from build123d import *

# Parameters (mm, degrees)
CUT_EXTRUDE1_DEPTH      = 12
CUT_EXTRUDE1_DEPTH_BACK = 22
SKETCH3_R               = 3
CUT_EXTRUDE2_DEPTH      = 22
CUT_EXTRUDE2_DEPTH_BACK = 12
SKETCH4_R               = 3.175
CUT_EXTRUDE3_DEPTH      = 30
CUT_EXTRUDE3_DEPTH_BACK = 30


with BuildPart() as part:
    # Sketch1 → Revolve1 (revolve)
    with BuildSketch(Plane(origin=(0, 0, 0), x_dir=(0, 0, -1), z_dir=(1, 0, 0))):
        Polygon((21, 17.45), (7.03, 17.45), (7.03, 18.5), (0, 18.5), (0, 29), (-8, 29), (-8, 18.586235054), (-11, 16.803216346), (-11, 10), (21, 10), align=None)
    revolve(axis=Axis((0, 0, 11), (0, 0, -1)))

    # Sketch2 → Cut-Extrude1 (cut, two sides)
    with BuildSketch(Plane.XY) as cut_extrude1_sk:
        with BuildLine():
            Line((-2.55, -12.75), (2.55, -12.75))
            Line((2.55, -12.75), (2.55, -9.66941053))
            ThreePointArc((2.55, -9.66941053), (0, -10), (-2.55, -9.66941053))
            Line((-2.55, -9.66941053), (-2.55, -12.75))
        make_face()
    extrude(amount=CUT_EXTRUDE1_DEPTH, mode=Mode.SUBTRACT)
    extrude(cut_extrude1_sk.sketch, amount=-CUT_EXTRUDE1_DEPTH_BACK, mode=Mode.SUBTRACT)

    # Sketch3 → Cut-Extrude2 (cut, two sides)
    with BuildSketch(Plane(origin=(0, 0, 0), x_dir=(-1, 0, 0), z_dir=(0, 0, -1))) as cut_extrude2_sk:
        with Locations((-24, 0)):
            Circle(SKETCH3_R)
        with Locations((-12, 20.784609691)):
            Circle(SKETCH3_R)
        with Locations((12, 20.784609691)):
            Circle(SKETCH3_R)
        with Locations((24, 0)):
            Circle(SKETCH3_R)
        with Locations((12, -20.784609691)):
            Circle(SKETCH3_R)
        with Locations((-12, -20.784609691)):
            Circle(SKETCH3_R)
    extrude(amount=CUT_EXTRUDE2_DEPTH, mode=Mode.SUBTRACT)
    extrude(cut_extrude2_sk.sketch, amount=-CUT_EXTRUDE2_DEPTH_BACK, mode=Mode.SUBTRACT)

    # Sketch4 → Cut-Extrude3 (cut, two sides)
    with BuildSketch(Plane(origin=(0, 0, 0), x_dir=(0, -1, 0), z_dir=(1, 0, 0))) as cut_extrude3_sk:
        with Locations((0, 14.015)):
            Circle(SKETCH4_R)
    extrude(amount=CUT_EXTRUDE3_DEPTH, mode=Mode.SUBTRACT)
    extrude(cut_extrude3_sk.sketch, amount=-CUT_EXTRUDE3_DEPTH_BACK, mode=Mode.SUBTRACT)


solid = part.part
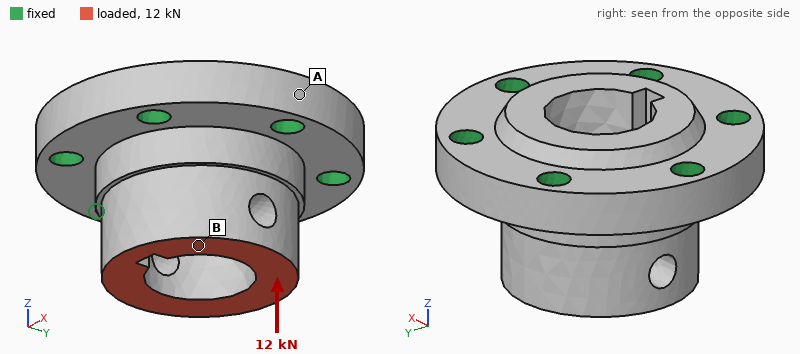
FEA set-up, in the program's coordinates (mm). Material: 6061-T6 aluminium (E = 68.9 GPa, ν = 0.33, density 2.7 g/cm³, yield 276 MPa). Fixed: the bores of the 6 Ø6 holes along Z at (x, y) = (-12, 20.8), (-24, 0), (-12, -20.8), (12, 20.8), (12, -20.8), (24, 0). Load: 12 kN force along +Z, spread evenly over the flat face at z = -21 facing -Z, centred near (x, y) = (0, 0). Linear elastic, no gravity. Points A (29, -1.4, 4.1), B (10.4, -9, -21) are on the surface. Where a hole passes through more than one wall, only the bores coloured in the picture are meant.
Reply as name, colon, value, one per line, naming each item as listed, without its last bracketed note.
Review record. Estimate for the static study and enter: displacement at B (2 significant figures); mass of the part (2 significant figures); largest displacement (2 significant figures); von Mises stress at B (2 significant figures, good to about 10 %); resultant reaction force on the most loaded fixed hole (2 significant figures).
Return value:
displacement at B: 11 µm
mass of the part: 88 g
largest displacement: 15 µm
von Mises stress at B: 22 MPa
resultant reaction force on the most loaded fixed hole: 2.2 kN
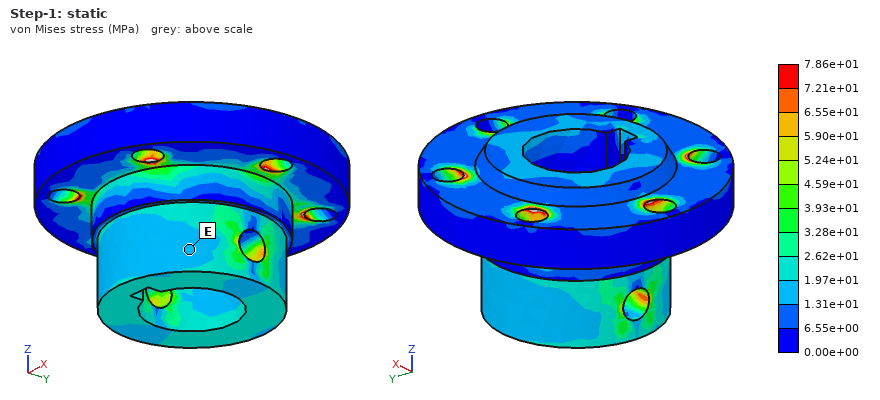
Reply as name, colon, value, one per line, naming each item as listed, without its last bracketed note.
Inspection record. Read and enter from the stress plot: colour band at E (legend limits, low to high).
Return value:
colour band at E: 1.31e+01 to 1.97e+01 MPa
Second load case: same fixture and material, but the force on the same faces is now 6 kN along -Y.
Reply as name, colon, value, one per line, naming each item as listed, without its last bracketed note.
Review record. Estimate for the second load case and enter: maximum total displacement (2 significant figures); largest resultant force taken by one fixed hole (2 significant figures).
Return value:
maximum total displacement: 35 µm
largest resultant force taken by one fixed hole: 2.4 kN
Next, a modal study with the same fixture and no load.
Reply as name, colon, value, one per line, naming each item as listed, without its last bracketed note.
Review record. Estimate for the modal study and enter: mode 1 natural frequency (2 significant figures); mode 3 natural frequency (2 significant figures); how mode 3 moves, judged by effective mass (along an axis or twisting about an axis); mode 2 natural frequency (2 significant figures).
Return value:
mode 1 natural frequency: 20 kHz
mode 3 natural frequency: 27 kHz
how mode 3 moves, judged by effective mass: along Z
mode 2 natural frequency: 21 kHz
